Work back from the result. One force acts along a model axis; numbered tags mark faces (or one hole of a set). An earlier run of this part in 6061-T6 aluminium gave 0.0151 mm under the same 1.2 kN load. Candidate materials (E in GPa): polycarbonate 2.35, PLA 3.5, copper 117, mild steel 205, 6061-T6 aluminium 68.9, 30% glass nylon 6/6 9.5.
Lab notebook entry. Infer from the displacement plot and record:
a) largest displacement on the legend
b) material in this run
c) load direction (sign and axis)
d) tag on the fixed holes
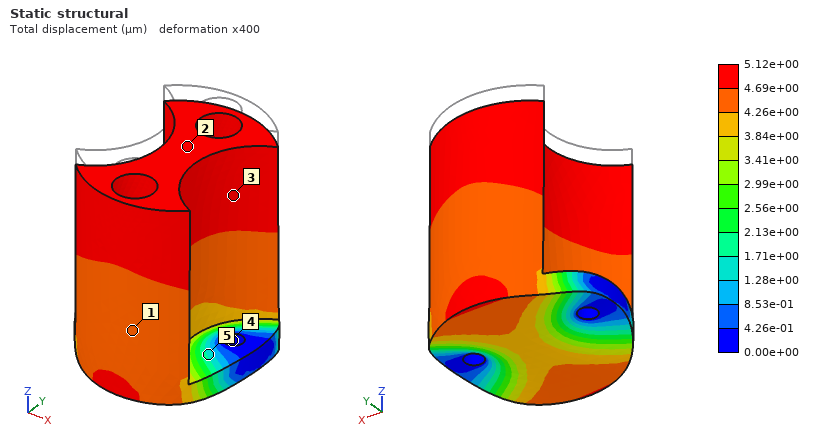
5.12e+00 µm
mild steel
-Z
4
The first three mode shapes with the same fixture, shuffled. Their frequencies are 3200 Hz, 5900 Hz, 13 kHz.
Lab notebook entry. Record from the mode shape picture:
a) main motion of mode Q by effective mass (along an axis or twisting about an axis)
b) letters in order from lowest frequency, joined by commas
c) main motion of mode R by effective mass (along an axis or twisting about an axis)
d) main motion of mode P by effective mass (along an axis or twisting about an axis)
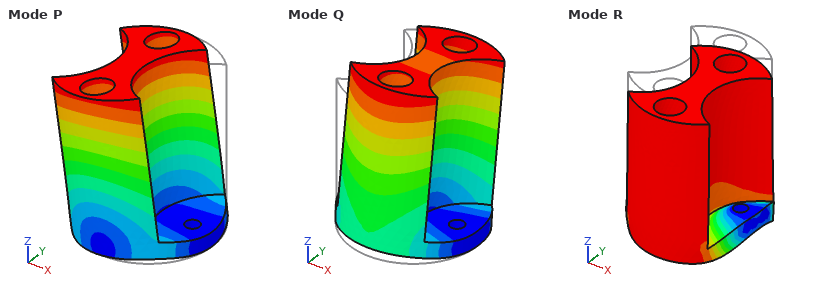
along Y
Q, P, R
along Z
along X
